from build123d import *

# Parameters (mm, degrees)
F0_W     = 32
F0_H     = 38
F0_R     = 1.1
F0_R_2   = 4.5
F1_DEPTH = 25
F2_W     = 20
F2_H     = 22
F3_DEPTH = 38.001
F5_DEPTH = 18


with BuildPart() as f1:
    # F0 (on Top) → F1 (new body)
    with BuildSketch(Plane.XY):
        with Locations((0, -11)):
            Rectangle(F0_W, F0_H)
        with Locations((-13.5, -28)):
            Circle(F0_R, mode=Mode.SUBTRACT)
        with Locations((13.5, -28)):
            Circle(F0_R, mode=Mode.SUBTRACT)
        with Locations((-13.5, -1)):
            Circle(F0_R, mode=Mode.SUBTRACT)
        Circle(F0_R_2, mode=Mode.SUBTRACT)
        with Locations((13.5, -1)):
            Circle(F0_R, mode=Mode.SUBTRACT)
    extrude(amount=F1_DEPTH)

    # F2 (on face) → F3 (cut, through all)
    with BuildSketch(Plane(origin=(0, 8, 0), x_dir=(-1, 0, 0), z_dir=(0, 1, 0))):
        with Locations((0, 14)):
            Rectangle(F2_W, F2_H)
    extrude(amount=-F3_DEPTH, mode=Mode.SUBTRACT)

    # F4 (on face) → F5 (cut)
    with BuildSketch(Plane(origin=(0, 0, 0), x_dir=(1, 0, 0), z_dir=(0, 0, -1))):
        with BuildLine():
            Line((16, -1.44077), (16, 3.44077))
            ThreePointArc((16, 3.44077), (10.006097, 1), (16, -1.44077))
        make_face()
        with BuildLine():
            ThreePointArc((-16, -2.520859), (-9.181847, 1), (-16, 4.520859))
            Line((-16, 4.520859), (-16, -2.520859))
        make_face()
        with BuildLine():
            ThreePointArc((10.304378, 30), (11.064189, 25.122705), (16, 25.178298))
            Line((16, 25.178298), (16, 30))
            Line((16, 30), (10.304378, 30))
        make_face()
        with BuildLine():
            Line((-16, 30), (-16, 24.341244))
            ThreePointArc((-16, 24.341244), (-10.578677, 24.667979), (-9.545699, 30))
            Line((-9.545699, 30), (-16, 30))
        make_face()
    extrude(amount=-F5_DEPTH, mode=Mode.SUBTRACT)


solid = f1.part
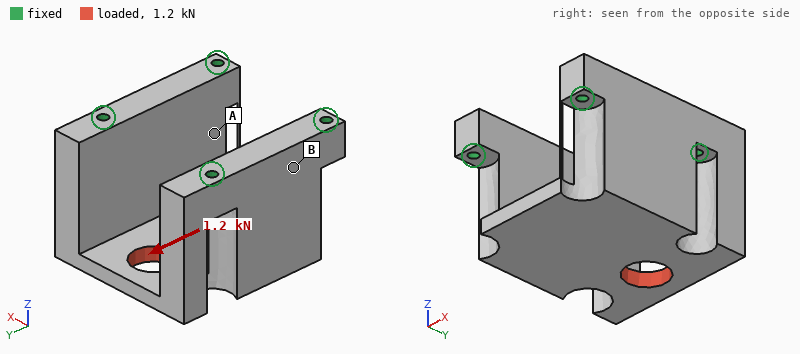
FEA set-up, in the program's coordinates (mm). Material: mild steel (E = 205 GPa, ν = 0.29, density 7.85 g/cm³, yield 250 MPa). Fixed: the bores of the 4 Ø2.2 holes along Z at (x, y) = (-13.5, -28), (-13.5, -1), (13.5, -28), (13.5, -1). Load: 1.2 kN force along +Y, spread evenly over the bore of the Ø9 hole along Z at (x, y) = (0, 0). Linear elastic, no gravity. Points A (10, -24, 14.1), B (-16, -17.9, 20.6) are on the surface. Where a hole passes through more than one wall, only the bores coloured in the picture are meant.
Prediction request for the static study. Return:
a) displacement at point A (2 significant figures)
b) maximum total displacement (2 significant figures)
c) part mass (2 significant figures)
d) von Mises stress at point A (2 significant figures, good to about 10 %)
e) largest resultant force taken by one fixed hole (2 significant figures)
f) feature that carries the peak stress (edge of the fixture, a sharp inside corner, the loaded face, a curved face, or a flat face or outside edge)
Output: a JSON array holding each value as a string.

["1.4 µm", "6.7 µm", "84 g", "19 MPa", "570 N", "a flat face or outside edge"]
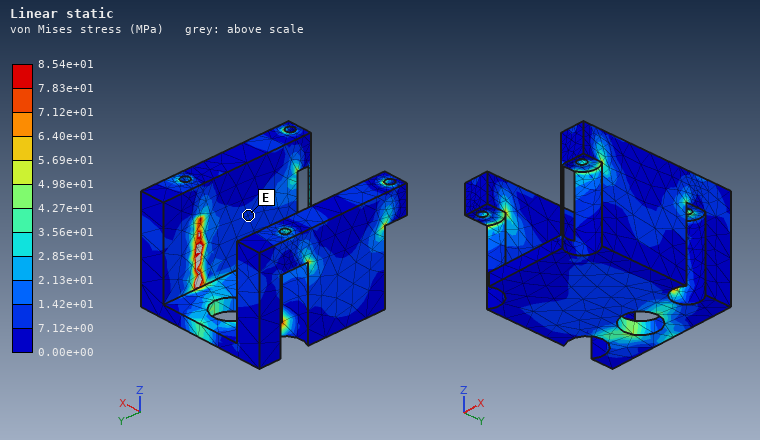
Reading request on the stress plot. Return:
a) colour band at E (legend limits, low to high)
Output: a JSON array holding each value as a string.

["7.12e+00 to 1.42e+01 MPa"]
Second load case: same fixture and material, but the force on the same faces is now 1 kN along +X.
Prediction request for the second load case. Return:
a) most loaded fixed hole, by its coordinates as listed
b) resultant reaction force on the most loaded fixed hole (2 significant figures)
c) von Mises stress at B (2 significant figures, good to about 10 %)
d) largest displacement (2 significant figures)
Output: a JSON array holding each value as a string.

["(13.5, -1)", "410 N", "16 MPa", "22 µm"]
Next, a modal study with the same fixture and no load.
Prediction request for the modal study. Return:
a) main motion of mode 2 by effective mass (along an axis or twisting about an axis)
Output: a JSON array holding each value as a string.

["along X"]
